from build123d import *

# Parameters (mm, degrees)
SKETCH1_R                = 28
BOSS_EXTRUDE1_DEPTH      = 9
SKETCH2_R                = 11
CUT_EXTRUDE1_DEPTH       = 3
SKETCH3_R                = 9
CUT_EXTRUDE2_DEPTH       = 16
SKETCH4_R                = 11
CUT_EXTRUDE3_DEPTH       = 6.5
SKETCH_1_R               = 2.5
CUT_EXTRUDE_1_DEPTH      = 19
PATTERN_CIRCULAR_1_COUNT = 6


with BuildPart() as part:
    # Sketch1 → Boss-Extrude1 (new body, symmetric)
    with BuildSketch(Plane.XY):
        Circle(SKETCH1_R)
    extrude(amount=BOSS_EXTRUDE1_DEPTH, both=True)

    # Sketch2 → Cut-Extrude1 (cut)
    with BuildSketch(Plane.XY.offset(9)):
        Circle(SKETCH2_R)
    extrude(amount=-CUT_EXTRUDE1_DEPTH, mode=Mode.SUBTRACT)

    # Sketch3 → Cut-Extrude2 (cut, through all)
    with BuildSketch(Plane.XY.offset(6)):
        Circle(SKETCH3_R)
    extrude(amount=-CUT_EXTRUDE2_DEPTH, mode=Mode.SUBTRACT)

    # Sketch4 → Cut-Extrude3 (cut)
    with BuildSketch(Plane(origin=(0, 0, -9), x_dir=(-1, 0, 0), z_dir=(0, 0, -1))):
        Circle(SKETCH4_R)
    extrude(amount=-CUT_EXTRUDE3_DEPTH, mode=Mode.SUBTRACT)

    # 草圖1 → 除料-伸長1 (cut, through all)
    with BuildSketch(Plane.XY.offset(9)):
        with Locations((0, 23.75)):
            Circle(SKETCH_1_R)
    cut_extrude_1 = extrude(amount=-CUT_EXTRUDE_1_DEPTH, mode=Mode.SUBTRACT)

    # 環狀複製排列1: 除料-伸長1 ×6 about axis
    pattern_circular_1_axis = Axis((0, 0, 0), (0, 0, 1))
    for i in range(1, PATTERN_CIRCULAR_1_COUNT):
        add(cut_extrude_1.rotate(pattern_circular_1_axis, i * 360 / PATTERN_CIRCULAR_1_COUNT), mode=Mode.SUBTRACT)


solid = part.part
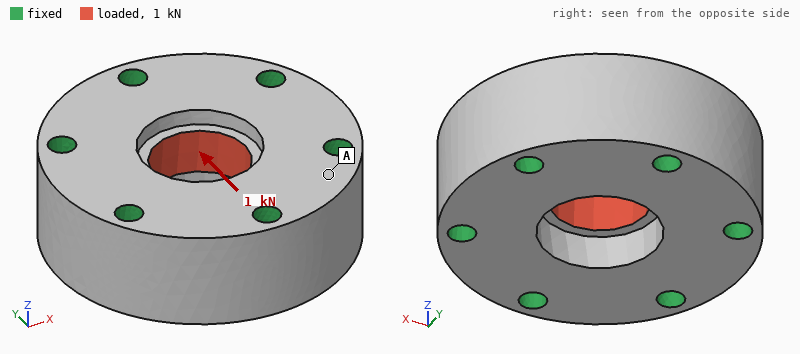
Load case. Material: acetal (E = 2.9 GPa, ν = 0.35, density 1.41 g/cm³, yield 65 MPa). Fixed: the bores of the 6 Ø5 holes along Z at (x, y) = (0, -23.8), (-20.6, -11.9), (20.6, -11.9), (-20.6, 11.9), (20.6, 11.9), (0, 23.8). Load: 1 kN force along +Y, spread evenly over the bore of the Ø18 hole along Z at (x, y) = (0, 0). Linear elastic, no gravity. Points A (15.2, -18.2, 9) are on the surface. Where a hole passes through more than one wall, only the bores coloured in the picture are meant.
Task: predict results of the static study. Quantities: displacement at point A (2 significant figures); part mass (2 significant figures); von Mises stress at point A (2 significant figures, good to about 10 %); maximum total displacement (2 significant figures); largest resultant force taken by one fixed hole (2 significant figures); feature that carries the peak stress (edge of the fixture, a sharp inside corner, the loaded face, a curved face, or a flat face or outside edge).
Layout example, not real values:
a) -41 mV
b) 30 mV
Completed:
a) 2.9 µm
b) 51 g
c) 0.44 MPa
d) 8.4 µm
e) 250 N
f) a sharp inside corner
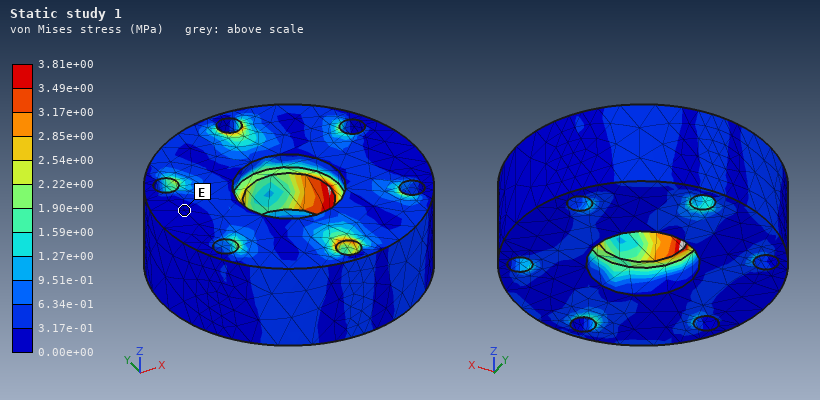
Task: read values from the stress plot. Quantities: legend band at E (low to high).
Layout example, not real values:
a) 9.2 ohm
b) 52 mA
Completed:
a) 0.00e+00 to 3.17e-01 MPa
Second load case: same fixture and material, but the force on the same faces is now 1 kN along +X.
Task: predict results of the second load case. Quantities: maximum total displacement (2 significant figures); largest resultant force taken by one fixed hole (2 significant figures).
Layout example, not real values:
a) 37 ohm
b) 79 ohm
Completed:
a) 8.7 µm
b) 220 N
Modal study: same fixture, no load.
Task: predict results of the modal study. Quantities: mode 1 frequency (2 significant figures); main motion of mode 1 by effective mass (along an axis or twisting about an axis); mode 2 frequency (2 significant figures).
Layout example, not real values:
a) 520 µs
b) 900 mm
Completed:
a) 13 kHz
b) along Z
c) 15 kHz
